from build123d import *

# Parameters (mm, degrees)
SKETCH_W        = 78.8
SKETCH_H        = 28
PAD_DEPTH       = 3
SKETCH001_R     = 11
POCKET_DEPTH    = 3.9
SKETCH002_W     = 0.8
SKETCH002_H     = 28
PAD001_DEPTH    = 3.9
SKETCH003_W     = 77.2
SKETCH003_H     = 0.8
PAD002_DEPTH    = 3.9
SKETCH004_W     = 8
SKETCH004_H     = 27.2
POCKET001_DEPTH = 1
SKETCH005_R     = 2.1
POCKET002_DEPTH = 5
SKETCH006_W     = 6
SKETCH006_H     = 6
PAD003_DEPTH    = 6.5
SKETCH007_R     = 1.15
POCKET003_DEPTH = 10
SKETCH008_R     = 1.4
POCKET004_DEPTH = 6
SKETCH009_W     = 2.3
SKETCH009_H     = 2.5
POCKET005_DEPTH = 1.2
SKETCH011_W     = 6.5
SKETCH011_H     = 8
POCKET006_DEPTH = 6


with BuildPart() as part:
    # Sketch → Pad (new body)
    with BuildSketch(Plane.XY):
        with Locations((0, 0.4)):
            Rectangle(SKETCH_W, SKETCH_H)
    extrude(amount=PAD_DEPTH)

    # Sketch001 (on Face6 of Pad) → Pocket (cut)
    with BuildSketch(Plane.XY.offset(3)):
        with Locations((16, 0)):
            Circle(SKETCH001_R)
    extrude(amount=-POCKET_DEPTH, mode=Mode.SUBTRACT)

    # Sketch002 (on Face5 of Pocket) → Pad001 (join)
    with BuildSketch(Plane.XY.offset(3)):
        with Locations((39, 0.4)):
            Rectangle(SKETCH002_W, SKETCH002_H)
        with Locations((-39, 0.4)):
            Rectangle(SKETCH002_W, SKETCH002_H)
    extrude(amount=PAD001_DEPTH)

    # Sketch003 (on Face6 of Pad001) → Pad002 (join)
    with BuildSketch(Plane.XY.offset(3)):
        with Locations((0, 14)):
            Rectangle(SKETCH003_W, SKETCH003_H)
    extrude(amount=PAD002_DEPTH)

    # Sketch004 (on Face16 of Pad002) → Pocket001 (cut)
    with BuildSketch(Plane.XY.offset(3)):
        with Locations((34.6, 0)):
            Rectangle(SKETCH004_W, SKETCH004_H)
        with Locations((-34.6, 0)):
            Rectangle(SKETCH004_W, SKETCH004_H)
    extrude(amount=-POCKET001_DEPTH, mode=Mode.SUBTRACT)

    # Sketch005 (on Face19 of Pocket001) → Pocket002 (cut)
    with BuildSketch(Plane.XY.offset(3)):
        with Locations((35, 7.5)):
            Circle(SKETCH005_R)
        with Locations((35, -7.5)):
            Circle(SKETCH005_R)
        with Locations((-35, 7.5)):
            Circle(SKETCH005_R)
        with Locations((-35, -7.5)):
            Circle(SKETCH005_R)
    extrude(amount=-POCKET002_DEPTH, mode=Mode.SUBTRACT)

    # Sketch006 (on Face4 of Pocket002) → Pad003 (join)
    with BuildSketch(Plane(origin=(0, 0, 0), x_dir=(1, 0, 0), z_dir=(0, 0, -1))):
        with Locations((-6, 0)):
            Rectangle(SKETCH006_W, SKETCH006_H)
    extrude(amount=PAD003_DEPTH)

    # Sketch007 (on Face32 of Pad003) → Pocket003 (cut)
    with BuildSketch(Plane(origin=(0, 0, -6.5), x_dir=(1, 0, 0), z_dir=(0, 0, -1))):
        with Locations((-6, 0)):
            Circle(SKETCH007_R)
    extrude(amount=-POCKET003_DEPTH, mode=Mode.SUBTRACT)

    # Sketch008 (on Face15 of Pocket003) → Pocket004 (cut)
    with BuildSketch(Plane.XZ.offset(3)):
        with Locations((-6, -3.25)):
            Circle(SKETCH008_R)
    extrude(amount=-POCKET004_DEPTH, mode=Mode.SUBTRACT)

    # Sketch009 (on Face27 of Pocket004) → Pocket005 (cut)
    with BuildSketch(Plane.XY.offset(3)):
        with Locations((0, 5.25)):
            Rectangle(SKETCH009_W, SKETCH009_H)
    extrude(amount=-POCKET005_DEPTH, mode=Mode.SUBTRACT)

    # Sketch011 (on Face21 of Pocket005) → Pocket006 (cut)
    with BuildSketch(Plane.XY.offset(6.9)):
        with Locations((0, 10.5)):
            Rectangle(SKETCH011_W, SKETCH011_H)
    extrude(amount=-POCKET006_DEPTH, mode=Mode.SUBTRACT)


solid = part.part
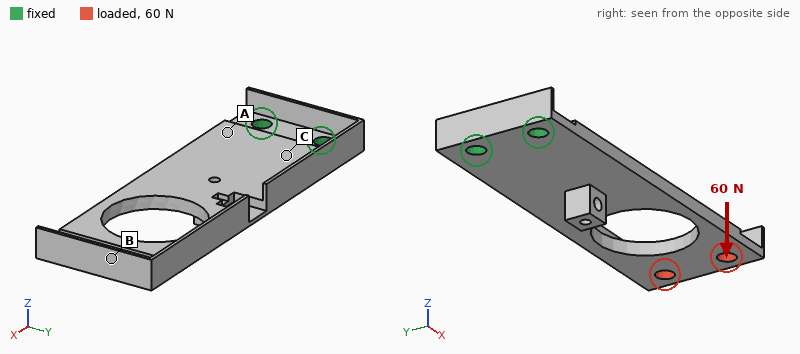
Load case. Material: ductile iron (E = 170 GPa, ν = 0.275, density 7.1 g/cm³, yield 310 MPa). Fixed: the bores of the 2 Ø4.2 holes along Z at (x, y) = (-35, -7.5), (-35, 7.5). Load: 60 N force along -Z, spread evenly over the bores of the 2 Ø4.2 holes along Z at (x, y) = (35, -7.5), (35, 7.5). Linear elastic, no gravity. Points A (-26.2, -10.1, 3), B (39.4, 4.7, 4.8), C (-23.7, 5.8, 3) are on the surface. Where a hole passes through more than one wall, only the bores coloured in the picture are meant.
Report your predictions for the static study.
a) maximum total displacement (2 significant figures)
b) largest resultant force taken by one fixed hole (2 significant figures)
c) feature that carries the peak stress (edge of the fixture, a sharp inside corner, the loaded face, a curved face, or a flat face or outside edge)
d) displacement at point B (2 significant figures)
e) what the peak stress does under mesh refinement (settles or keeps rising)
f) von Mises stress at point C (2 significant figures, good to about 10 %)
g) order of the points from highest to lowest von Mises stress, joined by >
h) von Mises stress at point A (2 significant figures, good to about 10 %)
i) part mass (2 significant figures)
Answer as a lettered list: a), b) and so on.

a) 0.88 mm
b) 95 N
c) edge of the fixture
d) 0.87 mm
e) keeps rising
f) 42 MPa
g) A > C > B
h) 64 MPa
i) 38 g
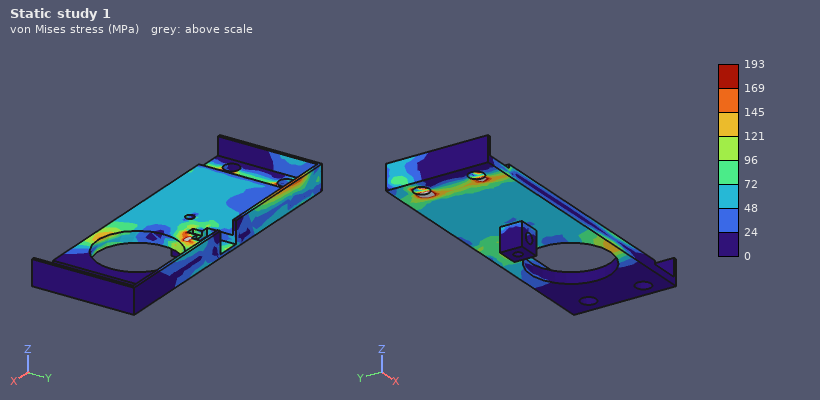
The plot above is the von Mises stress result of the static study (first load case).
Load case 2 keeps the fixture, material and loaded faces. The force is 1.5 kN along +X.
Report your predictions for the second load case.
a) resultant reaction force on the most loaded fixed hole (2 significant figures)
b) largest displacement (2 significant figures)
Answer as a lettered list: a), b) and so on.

a) 750 N
b) 0.15 mm
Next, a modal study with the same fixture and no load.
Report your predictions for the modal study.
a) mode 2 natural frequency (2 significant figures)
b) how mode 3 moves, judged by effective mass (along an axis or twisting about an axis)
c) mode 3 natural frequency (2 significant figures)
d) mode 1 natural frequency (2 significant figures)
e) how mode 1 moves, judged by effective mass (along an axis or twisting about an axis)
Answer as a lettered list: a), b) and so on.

a) 1900 Hz
b) along Z
c) 2200 Hz
d) 470 Hz
e) along Z
